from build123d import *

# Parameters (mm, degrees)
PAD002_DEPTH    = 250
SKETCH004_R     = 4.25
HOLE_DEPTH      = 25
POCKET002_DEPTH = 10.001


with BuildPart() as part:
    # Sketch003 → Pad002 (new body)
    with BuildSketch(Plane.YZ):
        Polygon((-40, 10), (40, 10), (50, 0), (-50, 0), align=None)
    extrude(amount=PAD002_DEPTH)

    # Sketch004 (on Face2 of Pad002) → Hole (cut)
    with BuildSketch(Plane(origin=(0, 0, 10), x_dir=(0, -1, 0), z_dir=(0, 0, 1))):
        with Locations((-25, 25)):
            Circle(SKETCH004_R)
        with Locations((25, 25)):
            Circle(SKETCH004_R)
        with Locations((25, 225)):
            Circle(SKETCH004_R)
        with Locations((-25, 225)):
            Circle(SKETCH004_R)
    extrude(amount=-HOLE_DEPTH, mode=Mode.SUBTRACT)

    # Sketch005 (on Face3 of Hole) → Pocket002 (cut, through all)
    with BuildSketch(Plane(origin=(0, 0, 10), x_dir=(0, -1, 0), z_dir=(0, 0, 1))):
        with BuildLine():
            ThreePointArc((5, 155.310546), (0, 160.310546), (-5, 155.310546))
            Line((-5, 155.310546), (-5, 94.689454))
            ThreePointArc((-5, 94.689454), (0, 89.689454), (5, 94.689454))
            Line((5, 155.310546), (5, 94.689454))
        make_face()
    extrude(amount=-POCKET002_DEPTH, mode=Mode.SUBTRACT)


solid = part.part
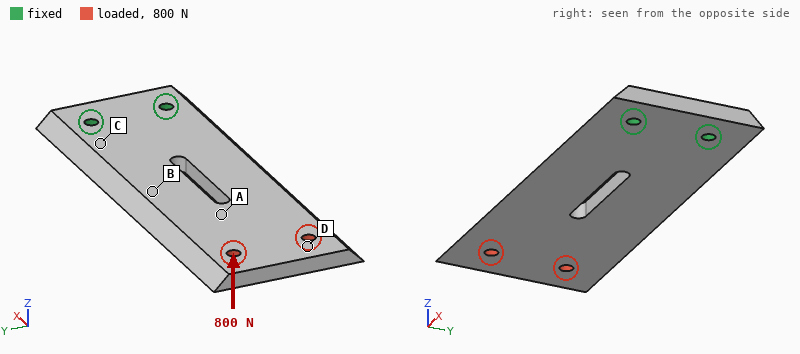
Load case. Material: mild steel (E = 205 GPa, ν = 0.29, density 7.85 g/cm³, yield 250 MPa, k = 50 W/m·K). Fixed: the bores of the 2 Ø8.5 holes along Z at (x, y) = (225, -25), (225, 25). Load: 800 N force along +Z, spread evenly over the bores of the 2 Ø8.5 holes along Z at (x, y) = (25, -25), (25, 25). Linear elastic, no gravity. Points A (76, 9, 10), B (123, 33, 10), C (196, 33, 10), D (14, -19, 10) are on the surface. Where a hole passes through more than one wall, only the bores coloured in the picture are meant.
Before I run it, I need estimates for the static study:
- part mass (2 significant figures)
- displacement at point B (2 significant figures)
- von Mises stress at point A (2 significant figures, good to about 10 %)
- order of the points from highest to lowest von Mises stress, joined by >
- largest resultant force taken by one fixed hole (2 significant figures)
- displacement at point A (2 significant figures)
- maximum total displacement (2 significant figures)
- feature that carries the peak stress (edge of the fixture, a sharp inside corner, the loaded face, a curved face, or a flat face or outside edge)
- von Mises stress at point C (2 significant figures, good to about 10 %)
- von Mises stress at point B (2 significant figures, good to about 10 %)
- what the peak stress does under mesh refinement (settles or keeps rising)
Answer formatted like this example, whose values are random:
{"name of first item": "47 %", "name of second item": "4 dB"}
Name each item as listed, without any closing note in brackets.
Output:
{"part mass": "1.7 kg", "displacement at point B": "0.47 mm", "von Mises stress at point A": "27 MPa", "order of the points from highest to lowest von Mises stress, joined by >": "C > B > A > D", "largest resultant force taken by one fixed hole": "420 N", "displacement at point A": "0.91 mm", "maximum total displacement": "1.7 mm", "feature that carries the peak stress": "edge of the fixture", "von Mises stress at point C": "95 MPa", "von Mises stress at point B": "61 MPa", "what the peak stress does under mesh refinement": "keeps rising"}
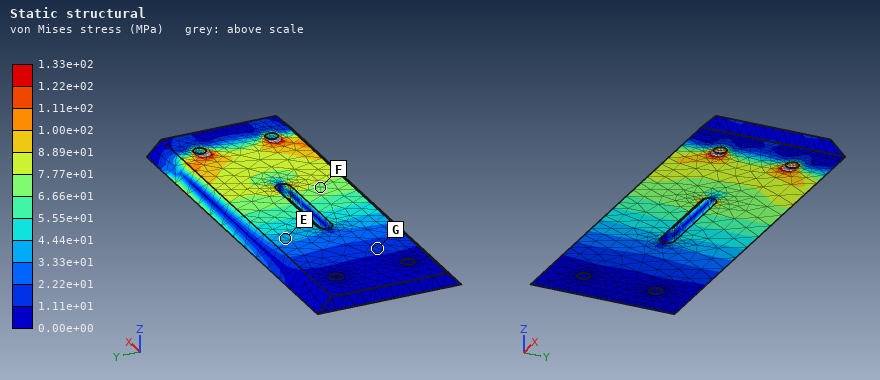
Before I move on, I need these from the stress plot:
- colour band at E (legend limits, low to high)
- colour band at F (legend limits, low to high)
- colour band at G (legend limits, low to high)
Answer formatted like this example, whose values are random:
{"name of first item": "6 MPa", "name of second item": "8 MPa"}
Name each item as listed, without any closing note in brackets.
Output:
{"colour band at E": "3.33e+01 to 4.44e+01 MPa", "colour band at F": "6.66e+01 to 7.77e+01 MPa", "colour band at G": "1.11e+01 to 2.22e+01 MPa"}
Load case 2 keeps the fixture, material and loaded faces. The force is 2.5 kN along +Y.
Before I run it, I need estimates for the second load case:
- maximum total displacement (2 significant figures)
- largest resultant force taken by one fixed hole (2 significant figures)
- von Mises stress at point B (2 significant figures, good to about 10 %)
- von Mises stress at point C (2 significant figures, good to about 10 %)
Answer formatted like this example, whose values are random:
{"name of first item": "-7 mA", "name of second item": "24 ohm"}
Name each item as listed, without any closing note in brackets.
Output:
{"maximum total displacement": "92 µm", "largest resultant force taken by one fixed hole": "9.3 kN", "von Mises stress at point B": "14 MPa", "von Mises stress at point C": "24 MPa"}
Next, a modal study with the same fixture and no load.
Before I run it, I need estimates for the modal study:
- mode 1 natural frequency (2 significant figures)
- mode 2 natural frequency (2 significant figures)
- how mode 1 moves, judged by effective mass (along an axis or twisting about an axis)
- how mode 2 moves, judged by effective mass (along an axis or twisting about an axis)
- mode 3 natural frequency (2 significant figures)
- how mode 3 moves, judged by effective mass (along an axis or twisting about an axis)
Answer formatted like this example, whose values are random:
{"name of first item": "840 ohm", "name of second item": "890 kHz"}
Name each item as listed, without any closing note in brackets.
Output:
{"mode 1 natural frequency": "160 Hz", "mode 2 natural frequency": "780 Hz", "how mode 1 moves, judged by effective mass": "along Z", "how mode 2 moves, judged by effective mass": "twisting about X", "mode 3 natural frequency": "1000 Hz", "how mode 3 moves, judged by effective mass": "along Z"}
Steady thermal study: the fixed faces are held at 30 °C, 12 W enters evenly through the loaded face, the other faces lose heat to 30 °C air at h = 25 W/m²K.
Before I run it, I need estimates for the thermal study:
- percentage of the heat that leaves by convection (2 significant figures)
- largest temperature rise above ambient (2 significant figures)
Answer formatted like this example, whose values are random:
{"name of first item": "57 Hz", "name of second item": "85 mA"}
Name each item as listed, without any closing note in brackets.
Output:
{"percentage of the heat that leaves by convection": "84 %", "largest temperature rise above ambient": "21 K"}
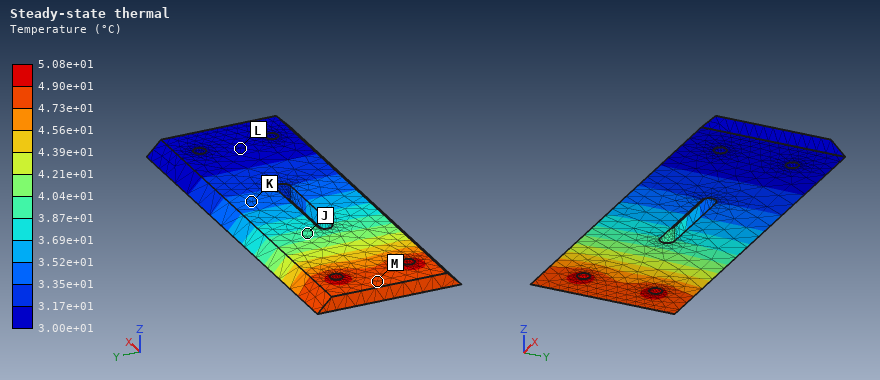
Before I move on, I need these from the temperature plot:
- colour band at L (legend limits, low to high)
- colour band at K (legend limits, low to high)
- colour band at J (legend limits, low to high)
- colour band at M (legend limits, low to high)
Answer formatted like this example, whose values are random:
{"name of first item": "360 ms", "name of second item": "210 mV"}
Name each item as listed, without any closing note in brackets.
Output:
{"colour band at L": "3.00e+01 to 3.17e+01 °C", "colour band at K": "3.35e+01 to 3.52e+01 °C", "colour band at J": "3.87e+01 to 4.04e+01 °C", "colour band at M": "4.73e+01 to 4.90e+01 °C"}
